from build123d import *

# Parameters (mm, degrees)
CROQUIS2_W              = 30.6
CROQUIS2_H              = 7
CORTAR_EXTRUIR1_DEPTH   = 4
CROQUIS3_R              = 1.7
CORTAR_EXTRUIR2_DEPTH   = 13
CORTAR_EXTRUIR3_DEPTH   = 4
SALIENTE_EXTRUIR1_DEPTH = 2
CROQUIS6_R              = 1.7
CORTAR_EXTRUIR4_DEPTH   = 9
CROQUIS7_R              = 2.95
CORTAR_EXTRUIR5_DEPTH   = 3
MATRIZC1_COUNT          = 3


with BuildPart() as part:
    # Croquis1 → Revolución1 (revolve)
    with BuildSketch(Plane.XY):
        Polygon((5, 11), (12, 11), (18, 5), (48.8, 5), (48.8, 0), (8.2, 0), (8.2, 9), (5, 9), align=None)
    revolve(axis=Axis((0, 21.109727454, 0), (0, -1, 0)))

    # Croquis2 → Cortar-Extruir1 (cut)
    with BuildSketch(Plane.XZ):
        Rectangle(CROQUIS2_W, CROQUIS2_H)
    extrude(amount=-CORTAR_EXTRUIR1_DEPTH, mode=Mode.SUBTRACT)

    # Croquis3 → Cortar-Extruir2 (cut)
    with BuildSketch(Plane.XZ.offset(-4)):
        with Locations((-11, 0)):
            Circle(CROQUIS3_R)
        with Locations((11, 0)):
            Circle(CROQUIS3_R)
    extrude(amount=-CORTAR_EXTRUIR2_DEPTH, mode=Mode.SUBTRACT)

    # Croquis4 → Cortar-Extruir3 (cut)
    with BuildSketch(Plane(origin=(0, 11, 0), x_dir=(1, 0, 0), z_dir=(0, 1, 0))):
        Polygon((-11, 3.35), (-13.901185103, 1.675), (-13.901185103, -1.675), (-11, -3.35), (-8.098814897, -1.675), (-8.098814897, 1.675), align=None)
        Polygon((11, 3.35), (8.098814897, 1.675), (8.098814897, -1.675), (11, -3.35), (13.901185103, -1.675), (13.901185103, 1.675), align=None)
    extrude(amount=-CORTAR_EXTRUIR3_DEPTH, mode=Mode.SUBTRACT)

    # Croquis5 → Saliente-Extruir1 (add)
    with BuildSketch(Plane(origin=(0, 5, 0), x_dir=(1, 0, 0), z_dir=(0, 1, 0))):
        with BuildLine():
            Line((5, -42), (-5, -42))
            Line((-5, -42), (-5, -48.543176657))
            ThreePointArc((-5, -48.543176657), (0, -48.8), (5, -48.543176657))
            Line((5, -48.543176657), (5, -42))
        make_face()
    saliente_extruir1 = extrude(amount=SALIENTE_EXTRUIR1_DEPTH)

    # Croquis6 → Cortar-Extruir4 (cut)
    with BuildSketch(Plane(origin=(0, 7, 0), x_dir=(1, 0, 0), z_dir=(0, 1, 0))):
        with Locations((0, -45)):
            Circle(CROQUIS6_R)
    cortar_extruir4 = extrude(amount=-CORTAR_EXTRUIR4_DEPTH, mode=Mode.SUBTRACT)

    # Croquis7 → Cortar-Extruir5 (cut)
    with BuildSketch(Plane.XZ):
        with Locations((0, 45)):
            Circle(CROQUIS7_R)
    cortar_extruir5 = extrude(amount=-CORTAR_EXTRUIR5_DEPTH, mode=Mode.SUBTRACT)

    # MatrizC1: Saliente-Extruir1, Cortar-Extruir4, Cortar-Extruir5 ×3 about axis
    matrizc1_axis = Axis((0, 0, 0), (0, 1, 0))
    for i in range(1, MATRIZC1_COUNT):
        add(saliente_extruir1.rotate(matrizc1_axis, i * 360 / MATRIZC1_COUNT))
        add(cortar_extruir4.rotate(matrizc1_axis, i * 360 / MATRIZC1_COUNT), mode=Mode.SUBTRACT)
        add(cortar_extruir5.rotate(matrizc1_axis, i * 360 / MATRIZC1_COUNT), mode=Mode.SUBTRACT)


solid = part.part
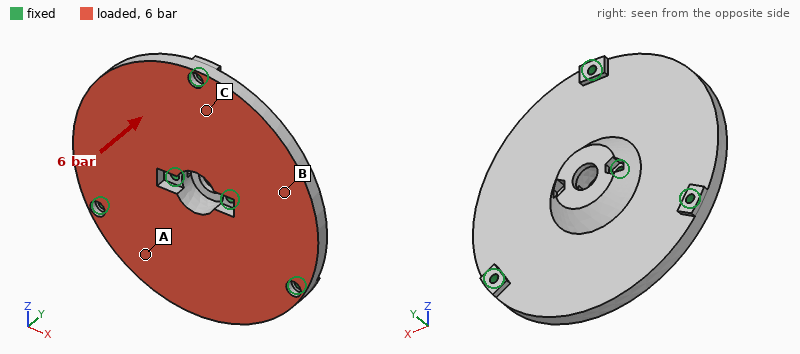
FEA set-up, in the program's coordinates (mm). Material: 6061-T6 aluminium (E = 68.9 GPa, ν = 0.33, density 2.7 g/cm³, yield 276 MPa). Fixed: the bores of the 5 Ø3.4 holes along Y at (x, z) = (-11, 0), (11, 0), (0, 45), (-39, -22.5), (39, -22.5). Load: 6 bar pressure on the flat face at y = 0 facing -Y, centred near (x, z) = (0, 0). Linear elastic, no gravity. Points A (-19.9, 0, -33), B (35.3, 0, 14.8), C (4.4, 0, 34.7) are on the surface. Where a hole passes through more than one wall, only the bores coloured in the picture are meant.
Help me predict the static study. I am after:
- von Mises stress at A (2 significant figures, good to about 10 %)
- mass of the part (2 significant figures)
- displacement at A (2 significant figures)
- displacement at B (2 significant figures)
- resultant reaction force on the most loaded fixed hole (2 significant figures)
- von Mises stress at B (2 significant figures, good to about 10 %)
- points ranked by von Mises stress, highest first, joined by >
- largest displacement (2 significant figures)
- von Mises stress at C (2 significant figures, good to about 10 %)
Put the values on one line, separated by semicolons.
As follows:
24 MPa; 110 g; 0.053 mm; 0.063 mm; 1.2 kN; 11 MPa; C > A > B; 0.13 mm; 40 MPa
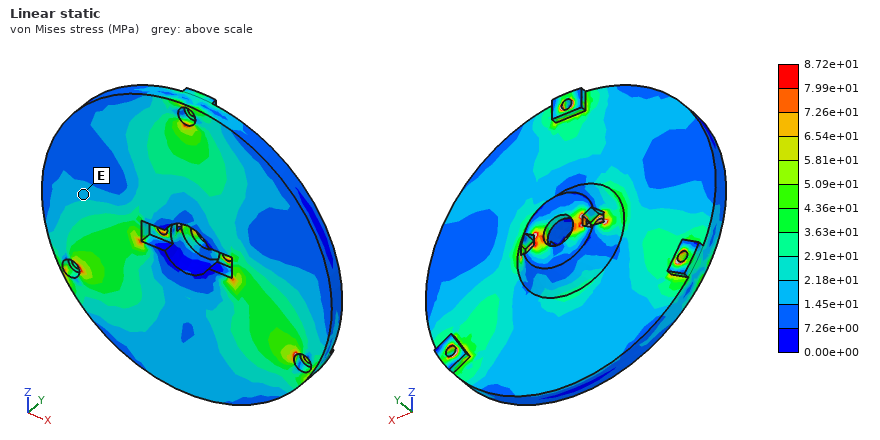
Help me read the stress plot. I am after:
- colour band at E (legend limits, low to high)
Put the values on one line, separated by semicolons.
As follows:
1.45e+01 to 2.18e+01 MPa
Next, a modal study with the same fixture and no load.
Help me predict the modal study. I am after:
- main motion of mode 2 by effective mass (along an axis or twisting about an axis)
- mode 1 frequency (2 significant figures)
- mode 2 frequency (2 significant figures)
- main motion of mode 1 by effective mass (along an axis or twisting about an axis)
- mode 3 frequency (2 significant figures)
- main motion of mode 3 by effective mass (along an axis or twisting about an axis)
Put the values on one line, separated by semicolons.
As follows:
twisting about Z; 3100 Hz; 3600 Hz; twisting about X; 4400 Hz; along Y
